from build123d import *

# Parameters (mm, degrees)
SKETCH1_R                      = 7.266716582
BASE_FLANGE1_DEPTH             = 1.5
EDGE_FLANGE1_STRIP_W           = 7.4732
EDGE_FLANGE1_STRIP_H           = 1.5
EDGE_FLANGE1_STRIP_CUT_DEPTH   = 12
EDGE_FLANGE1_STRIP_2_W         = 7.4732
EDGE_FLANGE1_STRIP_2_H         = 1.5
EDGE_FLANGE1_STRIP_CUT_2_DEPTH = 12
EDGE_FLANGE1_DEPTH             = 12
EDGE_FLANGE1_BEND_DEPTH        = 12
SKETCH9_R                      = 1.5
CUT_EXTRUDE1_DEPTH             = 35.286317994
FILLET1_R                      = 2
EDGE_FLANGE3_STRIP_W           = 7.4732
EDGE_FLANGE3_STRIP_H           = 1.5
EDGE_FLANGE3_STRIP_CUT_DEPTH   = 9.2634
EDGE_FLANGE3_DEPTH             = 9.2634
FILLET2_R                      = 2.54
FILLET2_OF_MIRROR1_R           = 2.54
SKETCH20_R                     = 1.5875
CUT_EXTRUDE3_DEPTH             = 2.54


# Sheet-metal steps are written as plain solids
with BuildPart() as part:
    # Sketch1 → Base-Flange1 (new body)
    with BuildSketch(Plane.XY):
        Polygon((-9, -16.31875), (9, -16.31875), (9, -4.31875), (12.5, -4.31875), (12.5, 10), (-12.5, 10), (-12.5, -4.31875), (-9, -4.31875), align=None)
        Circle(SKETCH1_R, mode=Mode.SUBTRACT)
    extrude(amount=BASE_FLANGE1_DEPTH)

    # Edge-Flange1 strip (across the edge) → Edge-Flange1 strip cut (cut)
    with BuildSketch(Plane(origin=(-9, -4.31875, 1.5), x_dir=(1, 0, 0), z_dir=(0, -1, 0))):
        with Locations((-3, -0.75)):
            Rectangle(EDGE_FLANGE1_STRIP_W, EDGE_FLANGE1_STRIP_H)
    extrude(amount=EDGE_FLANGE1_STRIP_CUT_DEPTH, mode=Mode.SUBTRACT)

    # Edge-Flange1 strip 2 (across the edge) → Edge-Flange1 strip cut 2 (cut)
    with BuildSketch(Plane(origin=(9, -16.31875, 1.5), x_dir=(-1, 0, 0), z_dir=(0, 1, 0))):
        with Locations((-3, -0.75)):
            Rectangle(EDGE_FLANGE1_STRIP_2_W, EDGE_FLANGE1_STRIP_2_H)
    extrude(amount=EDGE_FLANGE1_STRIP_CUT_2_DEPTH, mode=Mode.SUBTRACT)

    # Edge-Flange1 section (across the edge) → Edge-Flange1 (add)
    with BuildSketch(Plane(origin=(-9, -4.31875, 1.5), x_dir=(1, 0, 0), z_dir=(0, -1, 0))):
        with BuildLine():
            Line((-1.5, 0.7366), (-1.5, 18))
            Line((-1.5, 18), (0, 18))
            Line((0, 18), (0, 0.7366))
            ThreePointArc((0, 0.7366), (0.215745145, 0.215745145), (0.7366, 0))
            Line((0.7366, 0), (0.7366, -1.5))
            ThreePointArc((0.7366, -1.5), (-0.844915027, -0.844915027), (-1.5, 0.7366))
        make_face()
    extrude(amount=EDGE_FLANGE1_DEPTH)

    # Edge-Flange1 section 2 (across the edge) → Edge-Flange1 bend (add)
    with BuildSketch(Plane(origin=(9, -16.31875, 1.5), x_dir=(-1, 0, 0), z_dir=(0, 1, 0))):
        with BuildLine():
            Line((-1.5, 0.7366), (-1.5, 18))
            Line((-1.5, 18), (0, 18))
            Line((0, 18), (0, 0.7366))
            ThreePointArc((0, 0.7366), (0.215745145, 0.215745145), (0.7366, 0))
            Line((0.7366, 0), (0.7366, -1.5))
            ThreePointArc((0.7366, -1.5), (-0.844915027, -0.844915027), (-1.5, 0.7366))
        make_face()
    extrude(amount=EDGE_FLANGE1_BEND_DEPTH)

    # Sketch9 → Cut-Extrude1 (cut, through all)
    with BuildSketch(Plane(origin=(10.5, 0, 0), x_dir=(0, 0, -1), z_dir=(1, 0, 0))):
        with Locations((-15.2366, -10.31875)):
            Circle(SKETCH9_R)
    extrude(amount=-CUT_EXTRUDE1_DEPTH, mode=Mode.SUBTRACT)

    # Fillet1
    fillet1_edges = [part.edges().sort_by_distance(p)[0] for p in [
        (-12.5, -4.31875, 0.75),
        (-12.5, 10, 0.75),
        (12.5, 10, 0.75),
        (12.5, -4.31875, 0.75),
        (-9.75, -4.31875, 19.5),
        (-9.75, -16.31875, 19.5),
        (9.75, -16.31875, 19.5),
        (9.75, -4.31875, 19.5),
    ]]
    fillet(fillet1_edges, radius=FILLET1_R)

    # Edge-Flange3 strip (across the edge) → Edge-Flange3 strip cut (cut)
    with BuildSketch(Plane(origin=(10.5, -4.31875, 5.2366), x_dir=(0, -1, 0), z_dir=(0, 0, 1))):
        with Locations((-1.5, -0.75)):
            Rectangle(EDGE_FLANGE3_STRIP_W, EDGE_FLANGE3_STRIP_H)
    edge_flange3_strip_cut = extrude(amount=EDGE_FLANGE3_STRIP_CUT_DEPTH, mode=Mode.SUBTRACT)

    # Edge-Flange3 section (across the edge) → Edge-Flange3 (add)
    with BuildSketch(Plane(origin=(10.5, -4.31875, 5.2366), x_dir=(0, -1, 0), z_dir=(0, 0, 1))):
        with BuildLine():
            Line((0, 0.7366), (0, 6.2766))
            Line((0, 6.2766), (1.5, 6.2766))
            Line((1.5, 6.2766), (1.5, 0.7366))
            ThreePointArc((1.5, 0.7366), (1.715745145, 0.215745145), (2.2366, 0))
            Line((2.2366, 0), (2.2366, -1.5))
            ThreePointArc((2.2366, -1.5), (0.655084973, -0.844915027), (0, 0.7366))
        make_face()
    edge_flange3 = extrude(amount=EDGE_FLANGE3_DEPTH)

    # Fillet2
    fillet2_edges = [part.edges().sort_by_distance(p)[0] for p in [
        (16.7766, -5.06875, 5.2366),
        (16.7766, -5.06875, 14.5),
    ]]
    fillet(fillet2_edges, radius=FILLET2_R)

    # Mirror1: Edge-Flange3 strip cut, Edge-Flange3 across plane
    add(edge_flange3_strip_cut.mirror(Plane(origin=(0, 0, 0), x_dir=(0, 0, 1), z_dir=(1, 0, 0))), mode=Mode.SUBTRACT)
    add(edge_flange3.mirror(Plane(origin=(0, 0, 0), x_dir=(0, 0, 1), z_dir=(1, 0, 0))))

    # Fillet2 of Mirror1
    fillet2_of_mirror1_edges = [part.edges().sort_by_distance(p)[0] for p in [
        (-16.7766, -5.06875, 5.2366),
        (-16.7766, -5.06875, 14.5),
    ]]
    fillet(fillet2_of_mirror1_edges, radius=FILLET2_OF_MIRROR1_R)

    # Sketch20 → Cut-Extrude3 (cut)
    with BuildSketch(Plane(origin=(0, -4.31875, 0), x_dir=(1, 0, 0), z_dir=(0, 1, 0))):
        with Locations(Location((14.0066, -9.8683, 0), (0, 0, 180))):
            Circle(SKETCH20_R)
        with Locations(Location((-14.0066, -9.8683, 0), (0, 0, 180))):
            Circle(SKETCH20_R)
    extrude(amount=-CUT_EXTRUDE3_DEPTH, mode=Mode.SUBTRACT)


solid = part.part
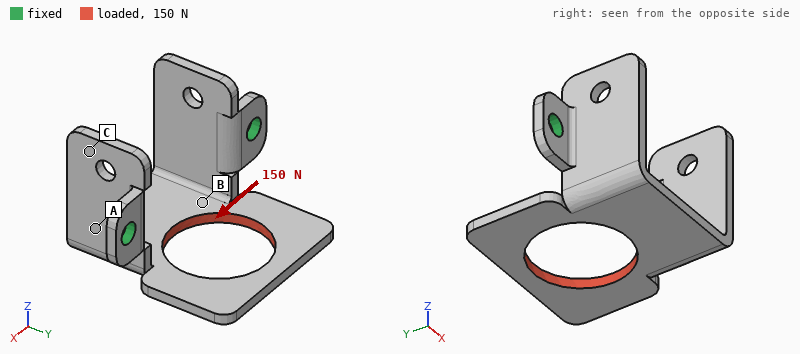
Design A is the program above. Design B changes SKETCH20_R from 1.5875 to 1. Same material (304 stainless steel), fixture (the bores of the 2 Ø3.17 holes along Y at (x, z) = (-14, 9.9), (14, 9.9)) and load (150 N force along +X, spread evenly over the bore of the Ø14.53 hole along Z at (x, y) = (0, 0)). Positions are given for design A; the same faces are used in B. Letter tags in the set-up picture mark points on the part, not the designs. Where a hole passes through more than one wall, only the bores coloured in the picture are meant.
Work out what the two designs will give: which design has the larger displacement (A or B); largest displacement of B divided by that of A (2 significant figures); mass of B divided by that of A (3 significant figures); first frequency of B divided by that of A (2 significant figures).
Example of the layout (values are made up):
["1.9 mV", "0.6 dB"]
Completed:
["B", "1.1", "1.01", "0.94"]
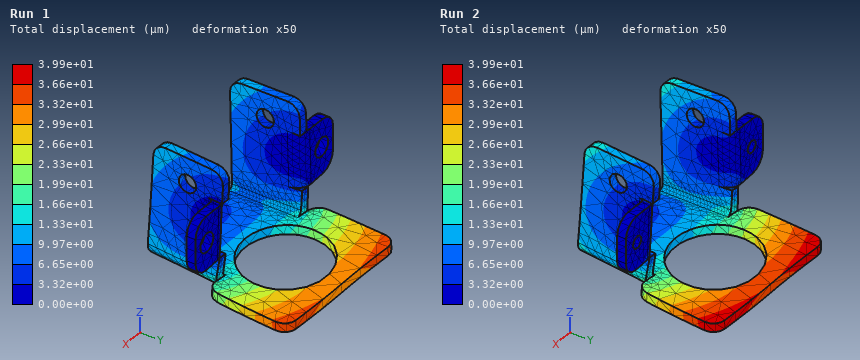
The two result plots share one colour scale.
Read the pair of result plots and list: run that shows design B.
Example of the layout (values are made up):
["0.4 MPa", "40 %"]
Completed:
["Run 2"]
